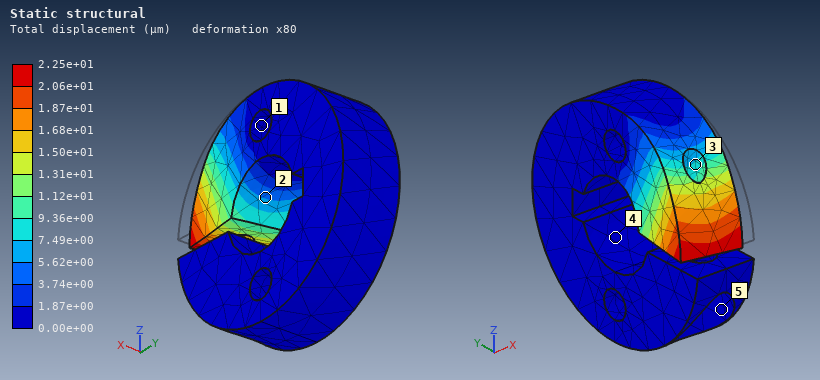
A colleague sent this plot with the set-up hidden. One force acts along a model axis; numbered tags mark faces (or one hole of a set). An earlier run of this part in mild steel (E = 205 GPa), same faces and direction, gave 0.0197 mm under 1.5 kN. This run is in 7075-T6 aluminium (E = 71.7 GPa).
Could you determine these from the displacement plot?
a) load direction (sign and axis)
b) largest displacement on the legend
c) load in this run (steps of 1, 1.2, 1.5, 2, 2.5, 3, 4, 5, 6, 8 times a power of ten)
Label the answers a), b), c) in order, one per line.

a) -X
b) 2.25e+01 µm
c) 600 N
